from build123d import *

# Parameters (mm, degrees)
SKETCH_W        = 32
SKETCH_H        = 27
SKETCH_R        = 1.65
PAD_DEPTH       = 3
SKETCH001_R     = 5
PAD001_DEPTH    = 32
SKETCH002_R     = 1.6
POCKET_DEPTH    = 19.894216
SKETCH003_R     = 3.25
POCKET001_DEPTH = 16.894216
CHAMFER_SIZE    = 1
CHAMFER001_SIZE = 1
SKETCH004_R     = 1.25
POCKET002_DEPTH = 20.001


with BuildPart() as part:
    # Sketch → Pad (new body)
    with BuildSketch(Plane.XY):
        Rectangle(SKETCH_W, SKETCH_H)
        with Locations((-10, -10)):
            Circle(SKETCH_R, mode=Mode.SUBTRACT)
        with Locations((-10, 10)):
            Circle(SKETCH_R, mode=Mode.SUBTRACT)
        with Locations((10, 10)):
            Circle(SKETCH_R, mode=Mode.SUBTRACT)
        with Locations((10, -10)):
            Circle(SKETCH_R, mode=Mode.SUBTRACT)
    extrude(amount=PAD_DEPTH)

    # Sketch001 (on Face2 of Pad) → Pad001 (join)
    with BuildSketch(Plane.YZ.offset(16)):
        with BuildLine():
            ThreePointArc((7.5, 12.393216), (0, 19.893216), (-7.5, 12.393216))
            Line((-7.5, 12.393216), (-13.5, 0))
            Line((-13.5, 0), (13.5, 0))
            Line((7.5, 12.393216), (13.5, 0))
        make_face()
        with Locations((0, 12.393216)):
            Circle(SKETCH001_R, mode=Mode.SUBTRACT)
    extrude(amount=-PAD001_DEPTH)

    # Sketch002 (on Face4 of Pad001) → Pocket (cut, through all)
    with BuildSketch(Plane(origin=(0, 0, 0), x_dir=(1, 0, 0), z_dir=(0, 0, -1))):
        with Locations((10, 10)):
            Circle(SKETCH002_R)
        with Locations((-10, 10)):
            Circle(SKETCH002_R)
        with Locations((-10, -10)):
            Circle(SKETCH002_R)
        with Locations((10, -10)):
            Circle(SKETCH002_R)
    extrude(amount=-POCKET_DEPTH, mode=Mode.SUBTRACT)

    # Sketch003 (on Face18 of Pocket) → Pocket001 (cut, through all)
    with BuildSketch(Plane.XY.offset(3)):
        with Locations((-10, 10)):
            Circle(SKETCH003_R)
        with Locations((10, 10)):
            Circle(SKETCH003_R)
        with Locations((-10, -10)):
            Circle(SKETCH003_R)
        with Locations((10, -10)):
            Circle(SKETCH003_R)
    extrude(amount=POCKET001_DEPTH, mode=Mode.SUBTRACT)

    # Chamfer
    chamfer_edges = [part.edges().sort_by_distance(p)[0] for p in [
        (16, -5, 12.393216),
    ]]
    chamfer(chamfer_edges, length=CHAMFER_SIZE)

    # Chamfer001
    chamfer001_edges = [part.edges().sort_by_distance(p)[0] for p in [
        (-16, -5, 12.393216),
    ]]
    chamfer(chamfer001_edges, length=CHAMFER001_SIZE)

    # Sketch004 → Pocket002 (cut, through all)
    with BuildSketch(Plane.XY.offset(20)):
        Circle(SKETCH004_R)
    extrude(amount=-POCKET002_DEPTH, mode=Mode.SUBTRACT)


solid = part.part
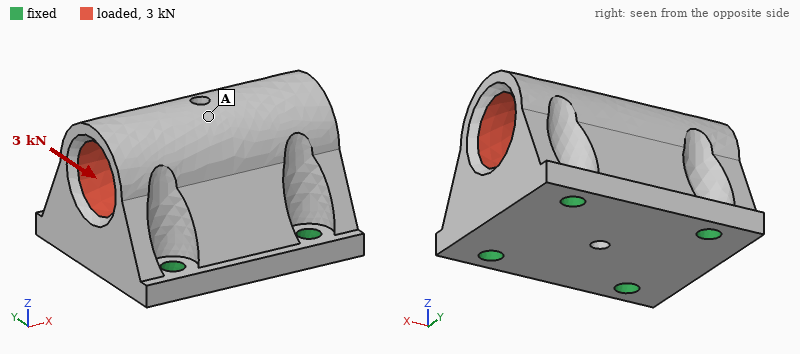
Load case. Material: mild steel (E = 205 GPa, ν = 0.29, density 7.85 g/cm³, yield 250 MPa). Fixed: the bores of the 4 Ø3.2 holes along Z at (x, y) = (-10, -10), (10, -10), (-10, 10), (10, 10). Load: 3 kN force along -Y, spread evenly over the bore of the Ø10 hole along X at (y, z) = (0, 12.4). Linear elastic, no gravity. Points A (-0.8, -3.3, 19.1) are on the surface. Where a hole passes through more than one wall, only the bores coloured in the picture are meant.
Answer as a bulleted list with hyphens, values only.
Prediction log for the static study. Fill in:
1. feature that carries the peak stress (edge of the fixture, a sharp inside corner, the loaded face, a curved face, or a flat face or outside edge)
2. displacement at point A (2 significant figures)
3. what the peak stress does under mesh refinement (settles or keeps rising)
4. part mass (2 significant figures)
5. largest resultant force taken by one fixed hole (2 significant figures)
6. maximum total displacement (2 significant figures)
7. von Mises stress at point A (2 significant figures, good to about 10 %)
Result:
- edge of the fixture
- 7.3 µm
- keeps rising
- 63 g
- 1.1 kN
- 7.4 µm
- 18 MPa
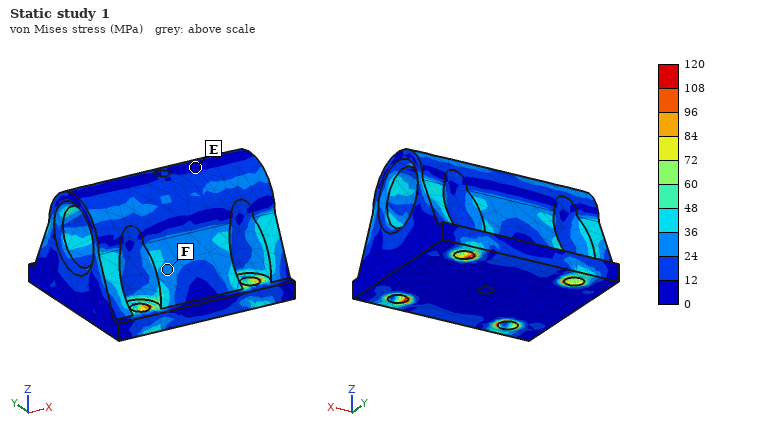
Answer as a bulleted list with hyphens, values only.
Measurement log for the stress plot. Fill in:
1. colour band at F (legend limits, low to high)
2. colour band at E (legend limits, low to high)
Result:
- 24 to 36 MPa
- 0 to 12 MPa
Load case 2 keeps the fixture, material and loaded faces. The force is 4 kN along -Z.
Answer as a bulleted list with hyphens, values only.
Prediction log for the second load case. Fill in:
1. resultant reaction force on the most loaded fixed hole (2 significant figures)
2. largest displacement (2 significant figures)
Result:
- 1.1 kN
- 3.1 µm
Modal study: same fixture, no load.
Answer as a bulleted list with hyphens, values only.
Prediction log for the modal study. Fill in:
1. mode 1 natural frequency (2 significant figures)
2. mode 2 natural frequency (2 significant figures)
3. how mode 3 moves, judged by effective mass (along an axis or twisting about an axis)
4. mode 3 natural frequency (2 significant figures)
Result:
- 22 kHz
- 23 kHz
- along Z
- 29 kHz
